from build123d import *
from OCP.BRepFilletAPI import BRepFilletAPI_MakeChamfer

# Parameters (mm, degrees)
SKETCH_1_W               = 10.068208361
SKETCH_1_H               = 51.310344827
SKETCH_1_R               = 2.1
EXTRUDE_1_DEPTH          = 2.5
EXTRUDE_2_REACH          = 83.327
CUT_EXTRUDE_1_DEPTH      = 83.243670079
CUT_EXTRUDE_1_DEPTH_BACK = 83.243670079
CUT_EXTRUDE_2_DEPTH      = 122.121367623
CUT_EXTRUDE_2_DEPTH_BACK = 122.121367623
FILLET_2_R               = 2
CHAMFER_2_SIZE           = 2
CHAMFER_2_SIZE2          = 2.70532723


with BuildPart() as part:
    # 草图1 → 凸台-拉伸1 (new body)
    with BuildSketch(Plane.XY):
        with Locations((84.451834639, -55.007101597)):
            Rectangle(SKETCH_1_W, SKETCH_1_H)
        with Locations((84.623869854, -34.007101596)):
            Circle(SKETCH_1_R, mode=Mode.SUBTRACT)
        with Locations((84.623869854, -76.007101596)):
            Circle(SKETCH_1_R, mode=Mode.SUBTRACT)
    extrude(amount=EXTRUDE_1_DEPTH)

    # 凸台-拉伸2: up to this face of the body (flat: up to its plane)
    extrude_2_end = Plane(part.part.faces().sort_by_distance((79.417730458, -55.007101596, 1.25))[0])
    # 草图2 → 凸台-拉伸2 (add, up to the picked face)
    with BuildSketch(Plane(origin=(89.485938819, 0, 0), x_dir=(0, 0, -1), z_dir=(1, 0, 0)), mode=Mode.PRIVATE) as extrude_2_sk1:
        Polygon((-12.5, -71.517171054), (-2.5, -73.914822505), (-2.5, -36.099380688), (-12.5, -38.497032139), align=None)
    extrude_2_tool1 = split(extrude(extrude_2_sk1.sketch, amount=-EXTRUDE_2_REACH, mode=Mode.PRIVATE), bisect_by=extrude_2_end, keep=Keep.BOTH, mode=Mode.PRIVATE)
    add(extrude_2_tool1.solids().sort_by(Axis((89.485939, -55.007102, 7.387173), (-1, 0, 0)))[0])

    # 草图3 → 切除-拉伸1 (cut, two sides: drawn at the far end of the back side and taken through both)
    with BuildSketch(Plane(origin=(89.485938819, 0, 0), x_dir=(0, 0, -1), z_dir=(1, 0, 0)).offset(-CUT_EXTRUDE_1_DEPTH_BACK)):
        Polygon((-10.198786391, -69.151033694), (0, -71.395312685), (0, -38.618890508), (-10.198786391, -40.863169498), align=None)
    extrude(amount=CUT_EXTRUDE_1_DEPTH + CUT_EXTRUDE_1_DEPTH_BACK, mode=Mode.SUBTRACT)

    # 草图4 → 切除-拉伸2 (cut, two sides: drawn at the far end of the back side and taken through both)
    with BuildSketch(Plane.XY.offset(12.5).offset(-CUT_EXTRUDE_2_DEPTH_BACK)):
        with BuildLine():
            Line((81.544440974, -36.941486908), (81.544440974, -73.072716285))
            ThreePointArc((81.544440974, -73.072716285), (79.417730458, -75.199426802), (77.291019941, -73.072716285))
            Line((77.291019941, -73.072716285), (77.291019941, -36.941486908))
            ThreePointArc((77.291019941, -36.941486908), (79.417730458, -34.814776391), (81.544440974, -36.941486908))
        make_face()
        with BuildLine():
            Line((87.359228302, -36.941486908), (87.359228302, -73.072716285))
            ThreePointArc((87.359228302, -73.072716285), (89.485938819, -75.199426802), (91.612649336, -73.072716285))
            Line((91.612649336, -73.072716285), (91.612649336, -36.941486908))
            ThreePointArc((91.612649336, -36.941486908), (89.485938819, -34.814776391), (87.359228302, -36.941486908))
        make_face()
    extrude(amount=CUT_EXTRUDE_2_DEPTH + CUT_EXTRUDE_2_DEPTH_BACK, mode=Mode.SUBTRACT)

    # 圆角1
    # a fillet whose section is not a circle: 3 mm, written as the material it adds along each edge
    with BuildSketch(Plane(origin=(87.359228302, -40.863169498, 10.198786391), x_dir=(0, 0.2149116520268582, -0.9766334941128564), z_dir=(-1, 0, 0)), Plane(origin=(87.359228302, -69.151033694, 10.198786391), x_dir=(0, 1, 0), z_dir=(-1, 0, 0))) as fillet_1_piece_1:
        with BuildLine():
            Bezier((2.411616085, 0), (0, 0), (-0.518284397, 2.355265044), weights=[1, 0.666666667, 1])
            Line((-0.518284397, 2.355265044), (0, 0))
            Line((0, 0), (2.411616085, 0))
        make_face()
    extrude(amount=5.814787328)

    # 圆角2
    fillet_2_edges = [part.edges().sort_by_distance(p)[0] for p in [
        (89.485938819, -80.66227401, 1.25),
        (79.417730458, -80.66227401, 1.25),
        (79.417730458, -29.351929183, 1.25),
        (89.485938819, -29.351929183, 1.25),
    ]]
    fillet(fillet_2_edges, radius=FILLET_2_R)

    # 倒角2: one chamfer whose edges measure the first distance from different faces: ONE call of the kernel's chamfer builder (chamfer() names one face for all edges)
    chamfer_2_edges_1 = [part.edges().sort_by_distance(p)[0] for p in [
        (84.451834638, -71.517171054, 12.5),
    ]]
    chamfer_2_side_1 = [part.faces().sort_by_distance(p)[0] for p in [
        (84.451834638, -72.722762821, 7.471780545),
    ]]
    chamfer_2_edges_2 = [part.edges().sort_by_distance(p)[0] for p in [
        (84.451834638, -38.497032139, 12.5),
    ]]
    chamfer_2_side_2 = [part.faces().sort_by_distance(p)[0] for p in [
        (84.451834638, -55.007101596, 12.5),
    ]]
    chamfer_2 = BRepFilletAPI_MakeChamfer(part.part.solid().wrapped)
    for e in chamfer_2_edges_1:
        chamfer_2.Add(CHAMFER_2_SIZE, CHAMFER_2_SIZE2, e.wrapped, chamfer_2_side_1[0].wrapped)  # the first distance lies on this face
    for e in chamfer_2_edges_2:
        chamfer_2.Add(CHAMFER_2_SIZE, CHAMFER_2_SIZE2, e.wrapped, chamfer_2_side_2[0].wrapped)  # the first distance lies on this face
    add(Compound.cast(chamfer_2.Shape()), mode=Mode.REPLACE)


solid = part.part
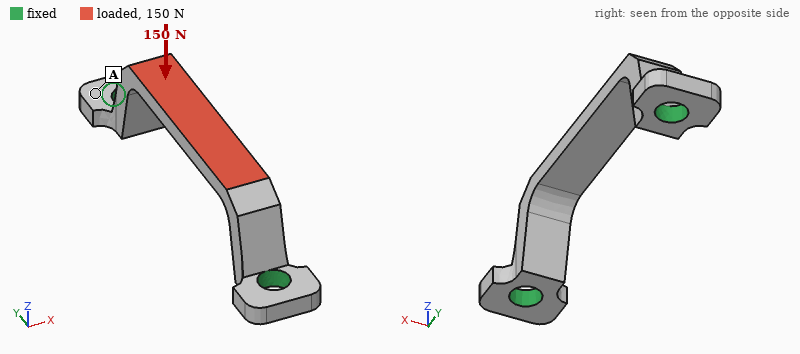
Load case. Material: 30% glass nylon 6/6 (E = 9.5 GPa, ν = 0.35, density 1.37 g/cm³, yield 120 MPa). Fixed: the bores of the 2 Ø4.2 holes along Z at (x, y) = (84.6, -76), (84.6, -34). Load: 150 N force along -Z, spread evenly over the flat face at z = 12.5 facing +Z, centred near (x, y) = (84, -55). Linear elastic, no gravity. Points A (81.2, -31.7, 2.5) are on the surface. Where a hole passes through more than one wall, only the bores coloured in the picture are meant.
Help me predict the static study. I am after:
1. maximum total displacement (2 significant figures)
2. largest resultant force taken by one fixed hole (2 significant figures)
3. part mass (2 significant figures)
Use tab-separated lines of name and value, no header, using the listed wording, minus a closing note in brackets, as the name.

maximum total displacement	0.23 mm
largest resultant force taken by one fixed hole	110 N
part mass	1.4 g
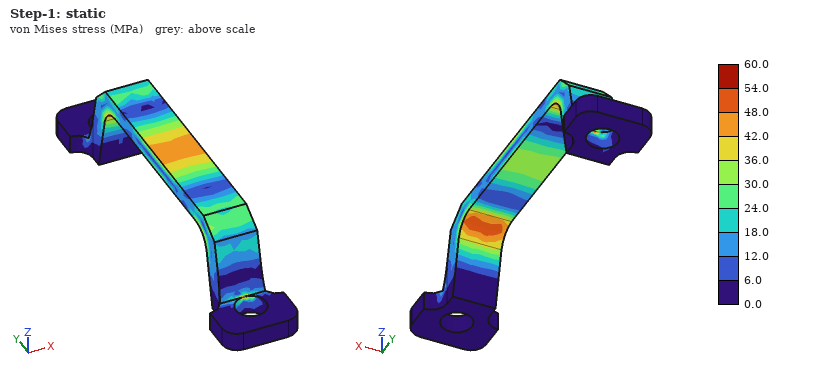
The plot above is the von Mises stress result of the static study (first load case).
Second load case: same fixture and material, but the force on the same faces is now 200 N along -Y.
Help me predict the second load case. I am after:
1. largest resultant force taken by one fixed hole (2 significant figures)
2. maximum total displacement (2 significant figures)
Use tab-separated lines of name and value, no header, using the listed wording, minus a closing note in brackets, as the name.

largest resultant force taken by one fixed hole	100 N
maximum total displacement	0.24 mm
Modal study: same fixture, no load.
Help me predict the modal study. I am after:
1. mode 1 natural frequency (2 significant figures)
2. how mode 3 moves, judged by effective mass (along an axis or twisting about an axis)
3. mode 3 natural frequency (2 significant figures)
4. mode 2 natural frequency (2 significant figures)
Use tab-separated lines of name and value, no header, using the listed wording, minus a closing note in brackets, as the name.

mode 1 natural frequency	5300 Hz
how mode 3 moves, judged by effective mass	along Z
mode 3 natural frequency	6400 Hz
mode 2 natural frequency	5500 Hz
